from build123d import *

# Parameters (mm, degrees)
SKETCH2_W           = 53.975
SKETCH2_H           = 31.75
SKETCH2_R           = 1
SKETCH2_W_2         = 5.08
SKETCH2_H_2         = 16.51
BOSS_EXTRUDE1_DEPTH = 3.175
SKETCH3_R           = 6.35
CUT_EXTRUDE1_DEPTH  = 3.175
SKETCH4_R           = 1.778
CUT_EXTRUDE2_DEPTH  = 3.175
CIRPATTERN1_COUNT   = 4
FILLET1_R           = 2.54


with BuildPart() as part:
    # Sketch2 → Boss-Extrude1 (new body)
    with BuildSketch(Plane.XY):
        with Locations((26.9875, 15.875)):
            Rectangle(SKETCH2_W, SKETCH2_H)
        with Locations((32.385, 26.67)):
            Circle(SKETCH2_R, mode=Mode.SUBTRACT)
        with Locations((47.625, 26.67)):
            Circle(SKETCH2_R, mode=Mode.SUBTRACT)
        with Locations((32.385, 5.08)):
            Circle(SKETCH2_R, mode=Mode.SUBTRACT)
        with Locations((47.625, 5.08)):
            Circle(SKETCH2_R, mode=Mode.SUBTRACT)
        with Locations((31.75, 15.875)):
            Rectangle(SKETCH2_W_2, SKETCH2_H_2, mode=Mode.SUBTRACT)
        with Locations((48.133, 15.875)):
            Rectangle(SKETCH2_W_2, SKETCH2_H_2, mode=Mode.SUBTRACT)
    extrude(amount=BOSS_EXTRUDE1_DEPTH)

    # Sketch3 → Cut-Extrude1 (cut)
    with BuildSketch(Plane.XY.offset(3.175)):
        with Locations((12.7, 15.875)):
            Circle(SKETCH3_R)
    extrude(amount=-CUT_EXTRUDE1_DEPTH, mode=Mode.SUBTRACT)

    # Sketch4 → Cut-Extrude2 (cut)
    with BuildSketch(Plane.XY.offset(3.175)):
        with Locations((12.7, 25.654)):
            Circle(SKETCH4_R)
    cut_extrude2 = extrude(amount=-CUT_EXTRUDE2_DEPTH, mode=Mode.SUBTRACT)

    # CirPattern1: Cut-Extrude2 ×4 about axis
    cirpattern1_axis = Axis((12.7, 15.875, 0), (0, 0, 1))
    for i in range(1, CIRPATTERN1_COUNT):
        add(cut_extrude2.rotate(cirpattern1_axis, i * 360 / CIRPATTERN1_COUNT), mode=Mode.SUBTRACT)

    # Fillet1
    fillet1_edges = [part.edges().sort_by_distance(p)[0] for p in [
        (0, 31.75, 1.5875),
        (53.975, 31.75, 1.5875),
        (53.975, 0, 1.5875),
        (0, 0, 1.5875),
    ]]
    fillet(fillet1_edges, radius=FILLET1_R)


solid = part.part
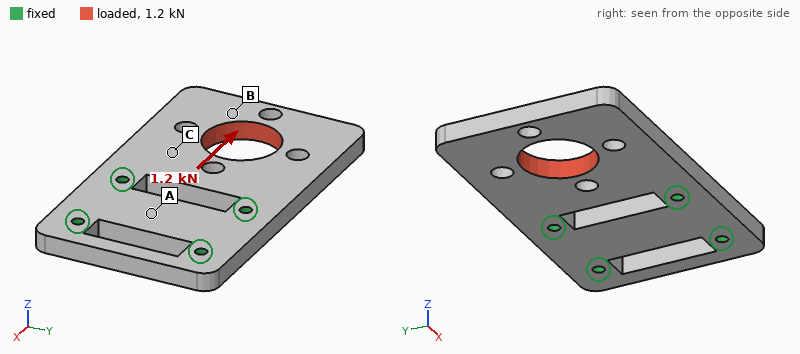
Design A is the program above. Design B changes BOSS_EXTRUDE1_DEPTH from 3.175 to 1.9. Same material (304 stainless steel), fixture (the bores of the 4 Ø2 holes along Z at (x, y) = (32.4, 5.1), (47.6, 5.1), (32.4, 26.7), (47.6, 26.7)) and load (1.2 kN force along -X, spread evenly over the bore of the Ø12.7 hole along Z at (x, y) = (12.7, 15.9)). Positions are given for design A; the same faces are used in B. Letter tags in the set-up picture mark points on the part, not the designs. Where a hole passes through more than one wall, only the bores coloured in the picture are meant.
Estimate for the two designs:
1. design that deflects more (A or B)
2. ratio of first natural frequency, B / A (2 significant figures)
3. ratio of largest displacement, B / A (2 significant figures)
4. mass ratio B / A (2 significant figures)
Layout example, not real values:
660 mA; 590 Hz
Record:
B; 0.62; 1.7; 0.60
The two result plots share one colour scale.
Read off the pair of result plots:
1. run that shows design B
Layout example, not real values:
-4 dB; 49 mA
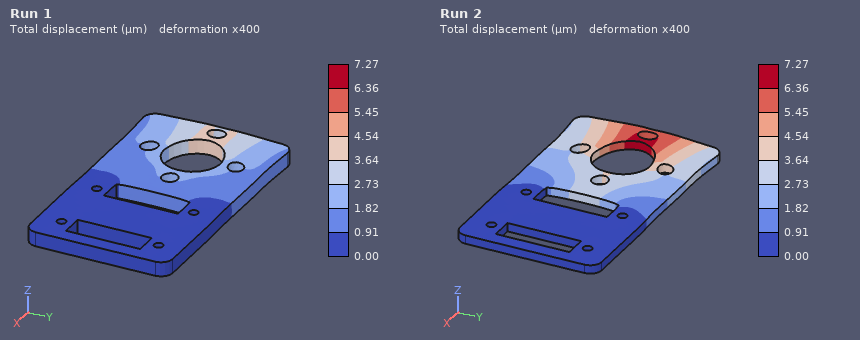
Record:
Run 2
